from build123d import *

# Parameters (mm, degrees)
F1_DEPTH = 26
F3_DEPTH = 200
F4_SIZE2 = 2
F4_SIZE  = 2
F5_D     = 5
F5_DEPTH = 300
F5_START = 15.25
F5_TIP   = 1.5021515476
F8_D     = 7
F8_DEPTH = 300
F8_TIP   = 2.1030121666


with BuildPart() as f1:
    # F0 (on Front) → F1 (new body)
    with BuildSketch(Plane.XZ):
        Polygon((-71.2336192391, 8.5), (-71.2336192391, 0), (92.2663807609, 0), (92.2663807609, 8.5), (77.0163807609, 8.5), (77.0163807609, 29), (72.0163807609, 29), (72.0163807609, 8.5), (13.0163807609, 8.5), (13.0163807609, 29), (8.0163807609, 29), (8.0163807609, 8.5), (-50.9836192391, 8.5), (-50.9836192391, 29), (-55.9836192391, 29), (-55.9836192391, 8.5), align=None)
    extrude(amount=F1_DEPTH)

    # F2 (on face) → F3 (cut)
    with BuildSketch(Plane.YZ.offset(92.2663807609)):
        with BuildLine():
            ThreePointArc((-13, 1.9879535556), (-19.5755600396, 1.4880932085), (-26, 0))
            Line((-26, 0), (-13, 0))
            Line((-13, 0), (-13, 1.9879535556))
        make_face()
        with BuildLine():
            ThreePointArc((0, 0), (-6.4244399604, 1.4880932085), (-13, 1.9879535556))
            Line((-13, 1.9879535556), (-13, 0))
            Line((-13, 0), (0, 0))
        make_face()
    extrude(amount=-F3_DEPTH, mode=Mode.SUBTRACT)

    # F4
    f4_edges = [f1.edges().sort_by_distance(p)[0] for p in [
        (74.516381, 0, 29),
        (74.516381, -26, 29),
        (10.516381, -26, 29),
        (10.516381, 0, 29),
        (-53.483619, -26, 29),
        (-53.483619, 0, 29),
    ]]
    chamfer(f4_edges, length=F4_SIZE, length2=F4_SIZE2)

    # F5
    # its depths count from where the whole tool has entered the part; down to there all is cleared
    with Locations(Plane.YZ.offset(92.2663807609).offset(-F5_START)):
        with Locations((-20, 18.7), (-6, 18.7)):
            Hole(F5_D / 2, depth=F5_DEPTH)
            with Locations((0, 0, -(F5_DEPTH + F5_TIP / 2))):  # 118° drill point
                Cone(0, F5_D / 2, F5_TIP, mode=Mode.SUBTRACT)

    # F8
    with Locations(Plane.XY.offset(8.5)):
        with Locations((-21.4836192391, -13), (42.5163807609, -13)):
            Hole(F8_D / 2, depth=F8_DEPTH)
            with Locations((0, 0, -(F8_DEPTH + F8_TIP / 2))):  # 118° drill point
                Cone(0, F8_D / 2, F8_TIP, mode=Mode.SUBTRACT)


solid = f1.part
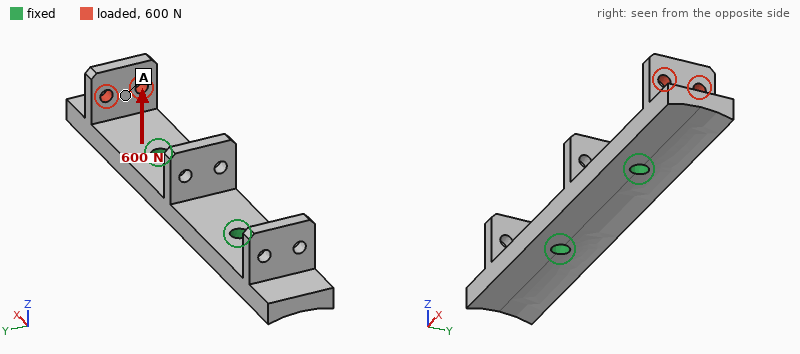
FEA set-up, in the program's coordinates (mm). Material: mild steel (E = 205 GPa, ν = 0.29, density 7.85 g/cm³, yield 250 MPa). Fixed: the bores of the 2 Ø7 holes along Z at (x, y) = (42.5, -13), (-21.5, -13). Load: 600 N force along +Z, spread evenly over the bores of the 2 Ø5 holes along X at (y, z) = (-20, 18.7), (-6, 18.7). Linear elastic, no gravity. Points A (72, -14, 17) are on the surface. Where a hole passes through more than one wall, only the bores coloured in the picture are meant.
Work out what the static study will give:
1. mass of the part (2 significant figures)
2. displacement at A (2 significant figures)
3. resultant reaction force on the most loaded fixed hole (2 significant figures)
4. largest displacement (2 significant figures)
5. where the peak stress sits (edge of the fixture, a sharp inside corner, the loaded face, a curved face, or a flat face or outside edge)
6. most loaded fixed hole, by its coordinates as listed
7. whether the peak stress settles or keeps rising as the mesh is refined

290 g
41 µm
640 N
71 µm
edge of the fixture
(42.5, -13)
keeps rising
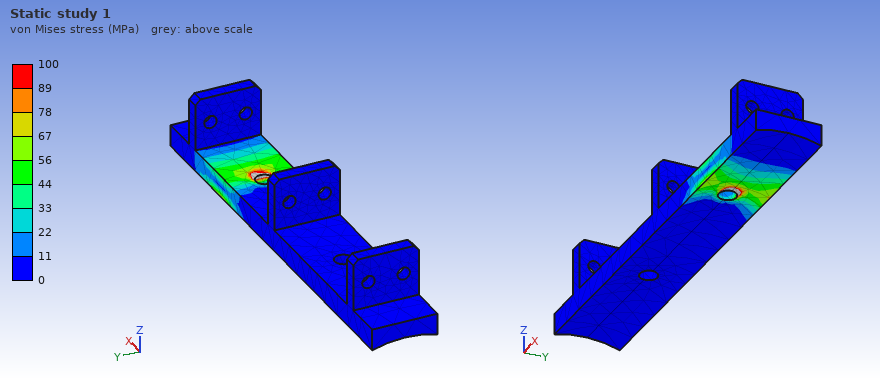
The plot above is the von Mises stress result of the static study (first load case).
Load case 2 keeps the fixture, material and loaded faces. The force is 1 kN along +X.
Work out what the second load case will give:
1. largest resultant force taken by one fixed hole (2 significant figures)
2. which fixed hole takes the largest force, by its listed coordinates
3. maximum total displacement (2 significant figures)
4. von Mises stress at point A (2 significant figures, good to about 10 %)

990 N
(42.5, -13)
97 µm
22 MPa
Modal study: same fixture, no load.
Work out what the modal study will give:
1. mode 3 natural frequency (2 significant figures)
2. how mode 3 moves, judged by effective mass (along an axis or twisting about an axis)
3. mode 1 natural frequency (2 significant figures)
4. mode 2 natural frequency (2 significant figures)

4200 Hz
along Y
2000 Hz
2000 Hz
